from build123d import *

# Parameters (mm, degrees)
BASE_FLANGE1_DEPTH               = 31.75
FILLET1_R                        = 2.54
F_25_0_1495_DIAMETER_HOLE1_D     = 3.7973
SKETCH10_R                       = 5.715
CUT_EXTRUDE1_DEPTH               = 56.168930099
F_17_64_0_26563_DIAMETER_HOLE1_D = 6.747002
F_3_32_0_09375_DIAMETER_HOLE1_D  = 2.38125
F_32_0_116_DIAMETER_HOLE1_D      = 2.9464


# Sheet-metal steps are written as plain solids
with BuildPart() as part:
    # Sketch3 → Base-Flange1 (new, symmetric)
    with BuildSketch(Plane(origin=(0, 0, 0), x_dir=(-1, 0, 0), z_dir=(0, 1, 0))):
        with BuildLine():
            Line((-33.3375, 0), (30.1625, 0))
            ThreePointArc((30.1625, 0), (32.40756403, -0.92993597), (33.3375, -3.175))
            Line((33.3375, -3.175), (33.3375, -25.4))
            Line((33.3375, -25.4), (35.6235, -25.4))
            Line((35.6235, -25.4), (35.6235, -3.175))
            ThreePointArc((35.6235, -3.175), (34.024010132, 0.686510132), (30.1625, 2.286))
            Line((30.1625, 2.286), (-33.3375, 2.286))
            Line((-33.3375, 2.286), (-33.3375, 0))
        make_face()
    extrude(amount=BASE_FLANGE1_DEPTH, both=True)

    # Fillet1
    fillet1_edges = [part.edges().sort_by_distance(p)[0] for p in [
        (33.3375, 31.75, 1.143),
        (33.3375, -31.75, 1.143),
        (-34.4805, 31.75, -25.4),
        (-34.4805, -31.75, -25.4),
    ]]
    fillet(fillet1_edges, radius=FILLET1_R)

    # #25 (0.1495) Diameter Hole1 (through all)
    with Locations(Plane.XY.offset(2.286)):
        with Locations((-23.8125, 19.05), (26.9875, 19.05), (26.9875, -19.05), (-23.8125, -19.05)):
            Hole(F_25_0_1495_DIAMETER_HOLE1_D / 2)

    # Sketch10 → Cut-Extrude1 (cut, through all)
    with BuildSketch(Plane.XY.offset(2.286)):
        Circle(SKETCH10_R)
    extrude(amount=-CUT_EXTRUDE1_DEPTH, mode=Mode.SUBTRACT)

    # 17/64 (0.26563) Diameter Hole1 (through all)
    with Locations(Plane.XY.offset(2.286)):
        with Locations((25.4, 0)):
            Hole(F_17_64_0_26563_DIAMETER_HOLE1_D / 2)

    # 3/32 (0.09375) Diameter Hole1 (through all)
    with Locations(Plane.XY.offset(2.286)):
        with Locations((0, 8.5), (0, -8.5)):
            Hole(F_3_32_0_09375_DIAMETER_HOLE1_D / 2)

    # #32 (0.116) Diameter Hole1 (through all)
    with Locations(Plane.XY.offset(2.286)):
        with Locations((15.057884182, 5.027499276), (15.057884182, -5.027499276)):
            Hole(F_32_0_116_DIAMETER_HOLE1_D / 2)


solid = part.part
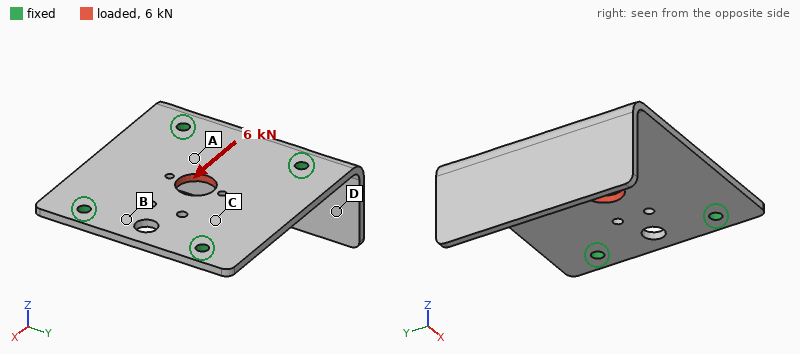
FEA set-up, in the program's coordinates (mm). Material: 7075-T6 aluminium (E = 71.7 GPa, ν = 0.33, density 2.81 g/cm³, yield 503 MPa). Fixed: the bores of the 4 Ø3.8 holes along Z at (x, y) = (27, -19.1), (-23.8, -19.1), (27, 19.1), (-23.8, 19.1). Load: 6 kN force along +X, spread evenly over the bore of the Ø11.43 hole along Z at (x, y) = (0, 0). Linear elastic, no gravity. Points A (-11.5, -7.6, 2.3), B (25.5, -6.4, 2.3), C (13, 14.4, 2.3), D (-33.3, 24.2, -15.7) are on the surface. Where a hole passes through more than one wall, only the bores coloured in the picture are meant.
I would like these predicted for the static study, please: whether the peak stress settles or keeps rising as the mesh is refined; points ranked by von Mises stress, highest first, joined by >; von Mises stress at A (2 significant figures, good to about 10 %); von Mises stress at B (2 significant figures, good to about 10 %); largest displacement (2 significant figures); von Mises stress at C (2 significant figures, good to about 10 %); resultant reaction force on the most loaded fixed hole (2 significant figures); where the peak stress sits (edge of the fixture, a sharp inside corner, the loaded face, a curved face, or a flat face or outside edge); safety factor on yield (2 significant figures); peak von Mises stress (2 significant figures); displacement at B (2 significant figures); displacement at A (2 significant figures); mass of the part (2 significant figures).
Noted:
settles
A > C > B > D
50 MPa
22 MPa
24 µm
36 MPa
1.7 kN
a flat face or outside edge
2.9
170 MPa
11 µm
14 µm
36 g
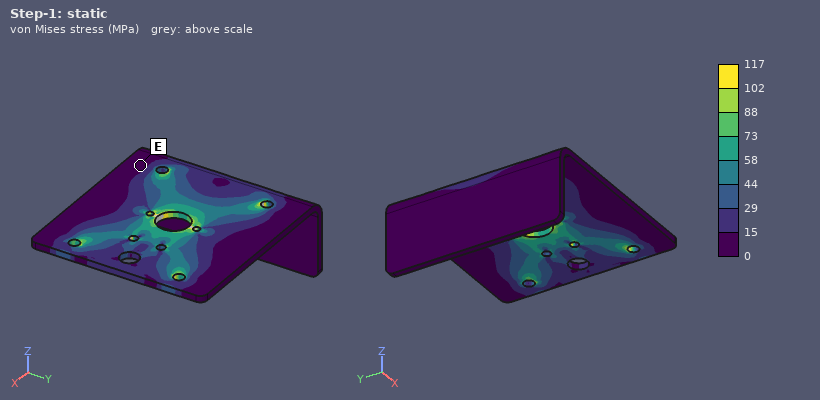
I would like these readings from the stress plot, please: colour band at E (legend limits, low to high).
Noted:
0 to 15 MPa
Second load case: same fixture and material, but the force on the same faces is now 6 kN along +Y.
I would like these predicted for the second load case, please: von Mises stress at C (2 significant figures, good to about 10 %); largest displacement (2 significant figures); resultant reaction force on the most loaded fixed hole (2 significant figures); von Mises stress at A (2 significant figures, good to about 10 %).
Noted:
43 MPa
33 µm
1.8 kN
53 MPa
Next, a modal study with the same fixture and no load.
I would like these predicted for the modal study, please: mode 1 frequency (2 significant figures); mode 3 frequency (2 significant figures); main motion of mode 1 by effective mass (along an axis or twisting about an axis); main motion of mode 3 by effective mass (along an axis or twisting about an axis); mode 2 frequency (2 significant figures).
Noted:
1700 Hz
4100 Hz
along X
along Z
2700 Hz
